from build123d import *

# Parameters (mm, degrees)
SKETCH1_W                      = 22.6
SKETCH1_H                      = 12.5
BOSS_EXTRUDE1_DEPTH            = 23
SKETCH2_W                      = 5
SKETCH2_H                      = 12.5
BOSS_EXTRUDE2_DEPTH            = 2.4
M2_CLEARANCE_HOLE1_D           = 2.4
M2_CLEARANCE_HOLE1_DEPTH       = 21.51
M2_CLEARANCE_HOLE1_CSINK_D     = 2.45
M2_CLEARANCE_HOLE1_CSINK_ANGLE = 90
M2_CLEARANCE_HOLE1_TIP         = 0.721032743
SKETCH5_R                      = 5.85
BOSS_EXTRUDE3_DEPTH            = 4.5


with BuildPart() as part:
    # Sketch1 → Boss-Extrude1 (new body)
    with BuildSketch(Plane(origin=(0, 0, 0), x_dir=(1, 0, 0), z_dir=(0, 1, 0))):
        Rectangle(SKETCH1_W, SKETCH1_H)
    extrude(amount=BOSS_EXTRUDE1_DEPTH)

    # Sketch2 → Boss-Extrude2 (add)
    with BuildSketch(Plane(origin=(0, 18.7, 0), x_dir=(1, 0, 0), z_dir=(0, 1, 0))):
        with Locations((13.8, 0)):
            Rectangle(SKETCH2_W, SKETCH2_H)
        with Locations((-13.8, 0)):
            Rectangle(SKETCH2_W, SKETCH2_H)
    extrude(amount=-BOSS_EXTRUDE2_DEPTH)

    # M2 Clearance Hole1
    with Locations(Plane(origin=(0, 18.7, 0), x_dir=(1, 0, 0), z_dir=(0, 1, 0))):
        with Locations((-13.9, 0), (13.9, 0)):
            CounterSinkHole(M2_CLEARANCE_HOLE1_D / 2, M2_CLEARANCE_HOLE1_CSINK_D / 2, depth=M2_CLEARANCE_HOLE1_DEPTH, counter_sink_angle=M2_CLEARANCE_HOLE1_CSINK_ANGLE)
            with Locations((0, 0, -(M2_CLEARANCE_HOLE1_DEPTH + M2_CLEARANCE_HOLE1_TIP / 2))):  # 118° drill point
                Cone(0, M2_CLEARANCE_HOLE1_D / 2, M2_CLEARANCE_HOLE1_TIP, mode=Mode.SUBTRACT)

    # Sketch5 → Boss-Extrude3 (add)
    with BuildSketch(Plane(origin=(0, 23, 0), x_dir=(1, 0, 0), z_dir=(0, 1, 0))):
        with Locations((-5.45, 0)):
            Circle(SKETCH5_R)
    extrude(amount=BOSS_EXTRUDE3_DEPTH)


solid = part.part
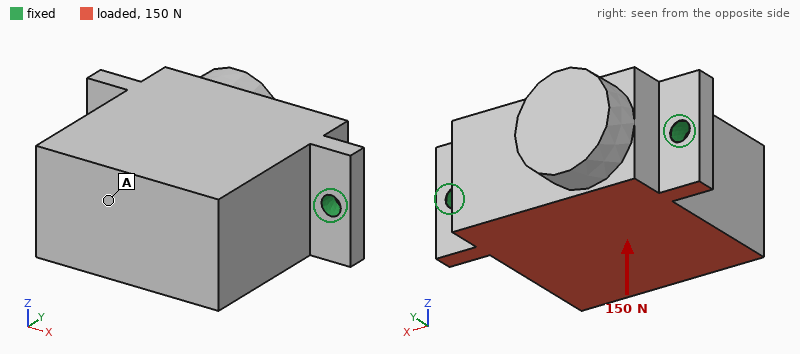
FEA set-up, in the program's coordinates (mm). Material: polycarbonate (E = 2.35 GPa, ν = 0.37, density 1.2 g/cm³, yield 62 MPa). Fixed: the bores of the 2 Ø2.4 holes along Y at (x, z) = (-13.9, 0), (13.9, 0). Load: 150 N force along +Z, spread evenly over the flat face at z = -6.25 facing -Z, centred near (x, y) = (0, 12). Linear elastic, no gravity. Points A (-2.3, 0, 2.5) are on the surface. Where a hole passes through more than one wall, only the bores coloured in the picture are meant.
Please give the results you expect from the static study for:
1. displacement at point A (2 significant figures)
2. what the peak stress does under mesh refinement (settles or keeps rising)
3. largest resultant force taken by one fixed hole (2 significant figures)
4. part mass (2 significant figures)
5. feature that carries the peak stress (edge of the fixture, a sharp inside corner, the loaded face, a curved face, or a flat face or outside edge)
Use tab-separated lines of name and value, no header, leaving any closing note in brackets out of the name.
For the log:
displacement at point A	0.46 mm
what the peak stress does under mesh refinement	keeps rising
largest resultant force taken by one fixed hole	75 N
part mass	8.7 g
feature that carries the peak stress	edge of the fixture
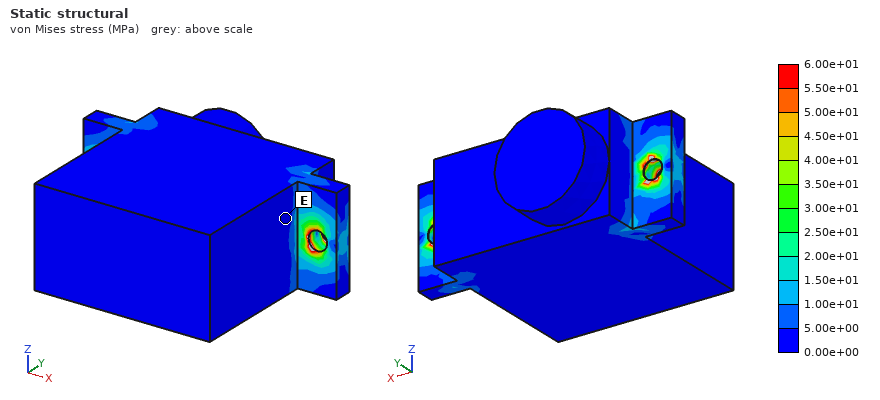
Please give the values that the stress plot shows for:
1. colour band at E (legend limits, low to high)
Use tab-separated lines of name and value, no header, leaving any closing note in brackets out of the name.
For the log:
colour band at E	0.00e+00 to 5.00e+00 MPa
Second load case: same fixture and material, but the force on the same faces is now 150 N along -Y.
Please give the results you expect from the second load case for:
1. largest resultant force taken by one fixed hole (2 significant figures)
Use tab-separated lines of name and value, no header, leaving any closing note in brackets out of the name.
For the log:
largest resultant force taken by one fixed hole	75 N
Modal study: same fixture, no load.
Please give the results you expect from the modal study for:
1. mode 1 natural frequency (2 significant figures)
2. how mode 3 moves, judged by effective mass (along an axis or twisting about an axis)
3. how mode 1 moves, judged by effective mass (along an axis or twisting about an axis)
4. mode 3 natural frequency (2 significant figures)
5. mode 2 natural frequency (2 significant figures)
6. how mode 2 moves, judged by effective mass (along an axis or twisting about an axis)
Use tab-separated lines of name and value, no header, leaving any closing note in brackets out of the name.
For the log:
mode 1 natural frequency	1100 Hz
how mode 3 moves, judged by effective mass	along X
how mode 1 moves, judged by effective mass	along Z
mode 3 natural frequency	4400 Hz
mode 2 natural frequency	4200 Hz
how mode 2 moves, judged by effective mass	along Y
